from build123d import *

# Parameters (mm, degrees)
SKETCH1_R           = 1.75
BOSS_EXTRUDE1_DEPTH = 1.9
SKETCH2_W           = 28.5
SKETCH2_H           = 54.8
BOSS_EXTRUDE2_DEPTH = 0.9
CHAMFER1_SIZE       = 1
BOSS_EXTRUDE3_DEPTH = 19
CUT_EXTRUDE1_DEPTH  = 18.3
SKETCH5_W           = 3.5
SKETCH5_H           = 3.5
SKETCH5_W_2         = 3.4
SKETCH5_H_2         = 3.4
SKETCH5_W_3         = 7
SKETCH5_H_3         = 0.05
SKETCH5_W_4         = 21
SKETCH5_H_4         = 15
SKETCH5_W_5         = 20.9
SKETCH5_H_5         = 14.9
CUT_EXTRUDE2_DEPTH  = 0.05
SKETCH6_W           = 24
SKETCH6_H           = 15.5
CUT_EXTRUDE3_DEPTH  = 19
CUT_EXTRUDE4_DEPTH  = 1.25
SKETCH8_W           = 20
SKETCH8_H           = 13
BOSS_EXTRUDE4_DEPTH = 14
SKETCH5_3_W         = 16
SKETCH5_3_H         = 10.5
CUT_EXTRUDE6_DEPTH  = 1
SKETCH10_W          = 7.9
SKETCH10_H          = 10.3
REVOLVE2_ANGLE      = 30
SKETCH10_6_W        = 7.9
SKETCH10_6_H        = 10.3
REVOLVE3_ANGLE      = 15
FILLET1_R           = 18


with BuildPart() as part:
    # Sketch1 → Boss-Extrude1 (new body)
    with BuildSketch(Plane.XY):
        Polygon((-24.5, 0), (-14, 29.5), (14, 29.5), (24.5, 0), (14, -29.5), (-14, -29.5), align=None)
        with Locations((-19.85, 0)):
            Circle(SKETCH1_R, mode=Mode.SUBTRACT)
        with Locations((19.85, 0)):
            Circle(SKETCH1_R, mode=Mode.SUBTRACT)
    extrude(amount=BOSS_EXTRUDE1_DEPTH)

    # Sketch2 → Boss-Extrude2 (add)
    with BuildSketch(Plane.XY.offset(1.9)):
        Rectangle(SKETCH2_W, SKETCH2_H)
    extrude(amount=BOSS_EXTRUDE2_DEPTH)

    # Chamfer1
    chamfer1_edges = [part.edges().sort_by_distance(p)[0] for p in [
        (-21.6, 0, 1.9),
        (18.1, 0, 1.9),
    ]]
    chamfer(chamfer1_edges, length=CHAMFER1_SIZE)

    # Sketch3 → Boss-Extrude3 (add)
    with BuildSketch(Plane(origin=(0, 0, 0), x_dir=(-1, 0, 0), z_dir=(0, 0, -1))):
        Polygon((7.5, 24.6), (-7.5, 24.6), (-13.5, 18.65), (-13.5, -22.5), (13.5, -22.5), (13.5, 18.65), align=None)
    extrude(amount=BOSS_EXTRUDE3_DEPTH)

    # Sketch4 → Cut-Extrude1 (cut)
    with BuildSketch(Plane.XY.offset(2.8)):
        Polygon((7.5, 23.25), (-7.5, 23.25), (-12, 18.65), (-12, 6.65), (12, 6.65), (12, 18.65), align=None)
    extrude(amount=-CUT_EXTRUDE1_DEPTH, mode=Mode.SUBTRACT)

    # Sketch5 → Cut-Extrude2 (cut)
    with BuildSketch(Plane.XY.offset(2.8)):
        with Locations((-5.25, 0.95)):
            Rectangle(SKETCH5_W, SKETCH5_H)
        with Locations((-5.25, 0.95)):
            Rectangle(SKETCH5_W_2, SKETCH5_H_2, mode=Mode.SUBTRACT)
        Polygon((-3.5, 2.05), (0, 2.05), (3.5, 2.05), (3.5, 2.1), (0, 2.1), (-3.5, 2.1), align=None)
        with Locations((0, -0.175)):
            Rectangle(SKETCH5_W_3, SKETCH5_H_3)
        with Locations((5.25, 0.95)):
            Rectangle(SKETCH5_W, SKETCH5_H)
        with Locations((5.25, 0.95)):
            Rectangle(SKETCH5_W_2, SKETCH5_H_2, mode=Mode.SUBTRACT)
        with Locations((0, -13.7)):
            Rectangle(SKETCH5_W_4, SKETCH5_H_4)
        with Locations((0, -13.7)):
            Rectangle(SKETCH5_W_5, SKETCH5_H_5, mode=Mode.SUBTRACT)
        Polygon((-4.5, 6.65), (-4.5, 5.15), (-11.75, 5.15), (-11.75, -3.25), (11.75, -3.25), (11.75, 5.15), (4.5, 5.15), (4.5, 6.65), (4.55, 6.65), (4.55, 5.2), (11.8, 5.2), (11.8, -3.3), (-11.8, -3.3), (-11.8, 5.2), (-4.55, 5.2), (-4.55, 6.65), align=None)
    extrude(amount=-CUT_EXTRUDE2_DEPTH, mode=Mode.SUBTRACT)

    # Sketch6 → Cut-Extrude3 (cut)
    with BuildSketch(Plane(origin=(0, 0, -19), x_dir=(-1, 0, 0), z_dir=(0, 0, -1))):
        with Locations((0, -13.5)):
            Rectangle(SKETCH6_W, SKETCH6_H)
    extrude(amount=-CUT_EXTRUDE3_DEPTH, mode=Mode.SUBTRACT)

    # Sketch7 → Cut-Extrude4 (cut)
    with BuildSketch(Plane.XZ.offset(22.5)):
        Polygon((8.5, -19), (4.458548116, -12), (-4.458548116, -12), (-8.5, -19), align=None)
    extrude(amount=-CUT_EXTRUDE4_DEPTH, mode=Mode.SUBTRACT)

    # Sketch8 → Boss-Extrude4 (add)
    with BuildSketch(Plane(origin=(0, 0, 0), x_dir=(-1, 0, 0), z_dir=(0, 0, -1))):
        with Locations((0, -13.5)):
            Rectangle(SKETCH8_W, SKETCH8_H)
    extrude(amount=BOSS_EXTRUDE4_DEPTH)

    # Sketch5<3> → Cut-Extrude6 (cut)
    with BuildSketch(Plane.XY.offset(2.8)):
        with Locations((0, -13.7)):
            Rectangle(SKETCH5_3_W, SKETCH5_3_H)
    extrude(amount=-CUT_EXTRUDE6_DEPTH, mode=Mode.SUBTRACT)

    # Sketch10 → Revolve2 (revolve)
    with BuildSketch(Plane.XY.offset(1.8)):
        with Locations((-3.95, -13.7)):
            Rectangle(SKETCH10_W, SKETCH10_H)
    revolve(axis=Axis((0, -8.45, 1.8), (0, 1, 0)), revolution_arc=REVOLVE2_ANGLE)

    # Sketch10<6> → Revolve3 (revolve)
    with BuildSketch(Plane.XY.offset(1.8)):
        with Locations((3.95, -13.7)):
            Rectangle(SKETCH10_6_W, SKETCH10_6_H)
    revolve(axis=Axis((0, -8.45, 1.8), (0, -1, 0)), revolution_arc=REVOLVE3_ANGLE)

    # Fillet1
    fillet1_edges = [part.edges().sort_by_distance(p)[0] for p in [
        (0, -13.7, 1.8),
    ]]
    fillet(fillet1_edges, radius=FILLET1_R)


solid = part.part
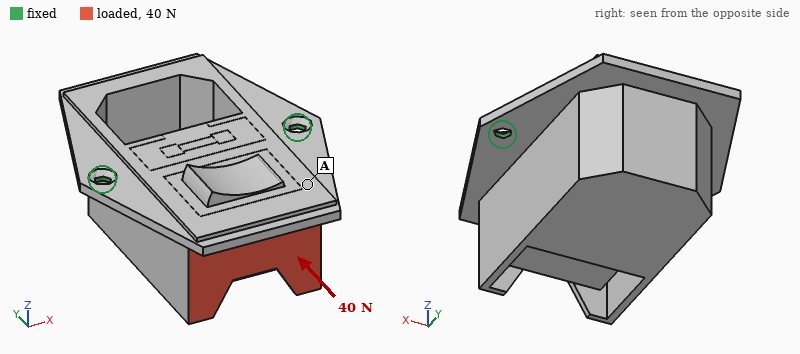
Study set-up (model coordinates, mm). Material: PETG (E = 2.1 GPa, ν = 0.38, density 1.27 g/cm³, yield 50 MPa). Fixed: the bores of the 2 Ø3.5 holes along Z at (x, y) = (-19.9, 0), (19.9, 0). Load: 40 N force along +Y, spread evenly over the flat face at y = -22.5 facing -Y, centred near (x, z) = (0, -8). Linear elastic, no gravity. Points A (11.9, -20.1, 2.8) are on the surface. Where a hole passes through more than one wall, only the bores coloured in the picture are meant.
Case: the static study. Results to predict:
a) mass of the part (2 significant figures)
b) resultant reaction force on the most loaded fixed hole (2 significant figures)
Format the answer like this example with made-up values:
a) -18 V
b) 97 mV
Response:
a) 24 g
b) 21 N
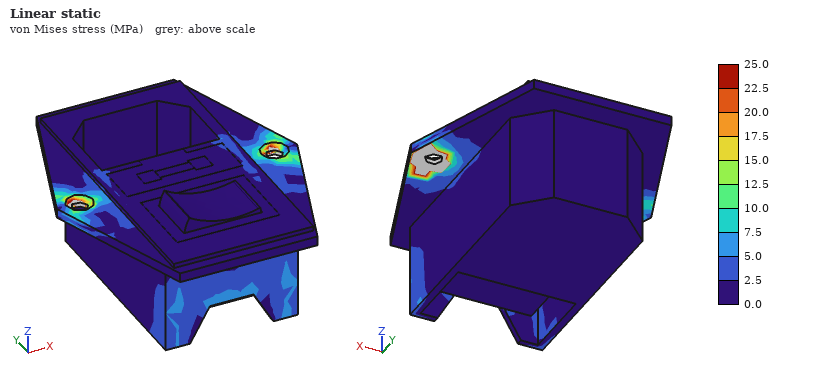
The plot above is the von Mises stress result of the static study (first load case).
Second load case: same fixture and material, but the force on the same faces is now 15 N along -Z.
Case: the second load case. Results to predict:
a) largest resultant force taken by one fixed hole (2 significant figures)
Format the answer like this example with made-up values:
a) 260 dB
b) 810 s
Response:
a) 8.2 N
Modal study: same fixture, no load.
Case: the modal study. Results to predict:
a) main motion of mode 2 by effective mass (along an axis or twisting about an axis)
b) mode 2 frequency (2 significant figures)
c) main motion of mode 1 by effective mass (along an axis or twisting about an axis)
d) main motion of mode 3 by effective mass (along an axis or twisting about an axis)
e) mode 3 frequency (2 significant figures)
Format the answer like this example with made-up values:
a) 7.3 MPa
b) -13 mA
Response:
a) along Z
b) 990 Hz
c) along Y
d) along X
e) 1200 Hz
